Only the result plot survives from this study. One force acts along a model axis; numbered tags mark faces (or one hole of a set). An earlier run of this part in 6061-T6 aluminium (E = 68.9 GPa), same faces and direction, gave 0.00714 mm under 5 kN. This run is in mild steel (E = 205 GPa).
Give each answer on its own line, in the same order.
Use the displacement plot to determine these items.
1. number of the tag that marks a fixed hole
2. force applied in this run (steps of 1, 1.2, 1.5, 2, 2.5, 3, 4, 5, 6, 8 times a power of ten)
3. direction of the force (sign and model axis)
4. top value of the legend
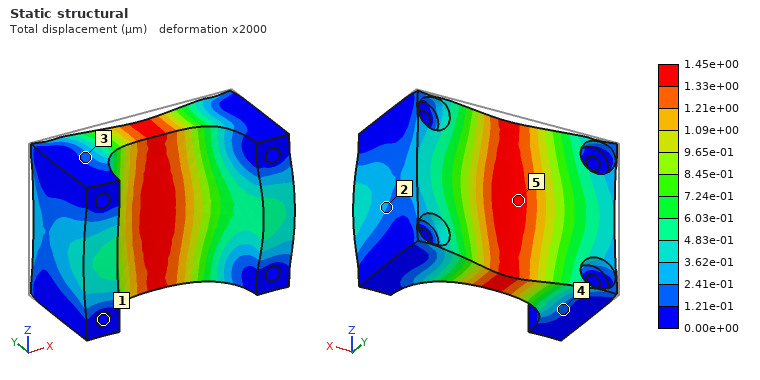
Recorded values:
1
3 kN
-Y
1.45e+00 µm
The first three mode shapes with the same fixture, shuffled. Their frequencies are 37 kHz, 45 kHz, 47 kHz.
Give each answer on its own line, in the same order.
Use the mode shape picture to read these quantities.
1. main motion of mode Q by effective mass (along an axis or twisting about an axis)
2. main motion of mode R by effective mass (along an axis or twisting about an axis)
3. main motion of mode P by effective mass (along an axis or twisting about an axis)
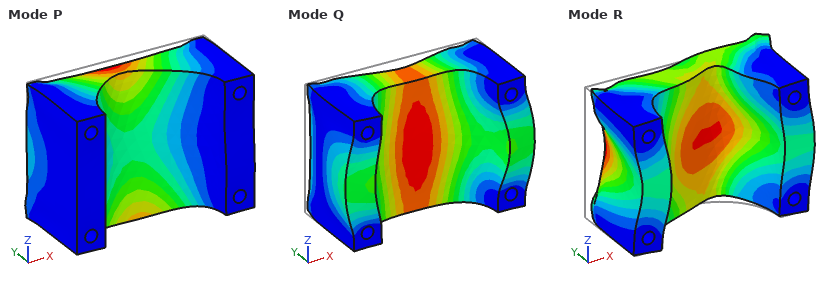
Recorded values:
along Y
along X
along Z
